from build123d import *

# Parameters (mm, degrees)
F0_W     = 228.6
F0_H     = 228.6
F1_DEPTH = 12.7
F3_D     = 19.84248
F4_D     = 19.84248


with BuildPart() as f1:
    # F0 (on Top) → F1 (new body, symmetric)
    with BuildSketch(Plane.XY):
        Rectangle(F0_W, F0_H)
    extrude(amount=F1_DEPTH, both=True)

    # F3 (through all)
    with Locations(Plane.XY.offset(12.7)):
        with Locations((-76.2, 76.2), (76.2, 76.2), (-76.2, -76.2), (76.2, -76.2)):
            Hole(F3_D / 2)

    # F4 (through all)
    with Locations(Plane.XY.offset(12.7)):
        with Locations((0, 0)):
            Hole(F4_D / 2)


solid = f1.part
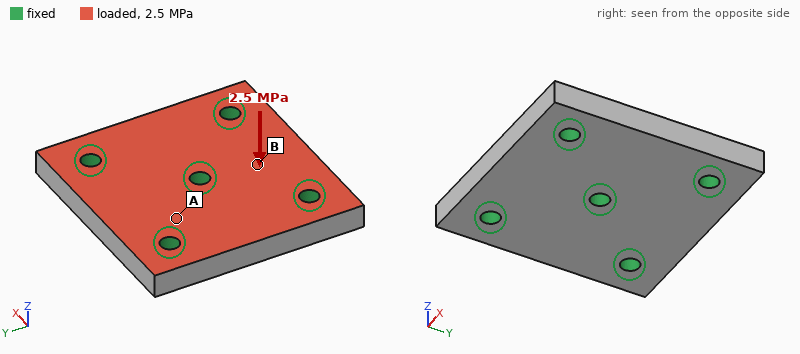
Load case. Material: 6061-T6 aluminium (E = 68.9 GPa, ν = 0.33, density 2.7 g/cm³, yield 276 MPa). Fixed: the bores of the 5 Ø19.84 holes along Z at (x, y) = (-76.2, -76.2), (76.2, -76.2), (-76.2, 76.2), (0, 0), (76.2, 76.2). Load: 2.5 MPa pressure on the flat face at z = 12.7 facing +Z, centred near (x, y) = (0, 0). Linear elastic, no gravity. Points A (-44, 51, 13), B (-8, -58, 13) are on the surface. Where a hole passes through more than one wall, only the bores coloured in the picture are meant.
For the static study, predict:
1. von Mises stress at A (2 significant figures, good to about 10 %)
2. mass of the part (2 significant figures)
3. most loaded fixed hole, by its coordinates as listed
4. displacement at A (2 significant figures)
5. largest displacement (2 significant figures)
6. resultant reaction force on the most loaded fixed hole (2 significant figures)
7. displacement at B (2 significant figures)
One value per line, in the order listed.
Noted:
17 MPa
3.5 kg
(0, 0)
17 µm
47 µm
28 kN
25 µm
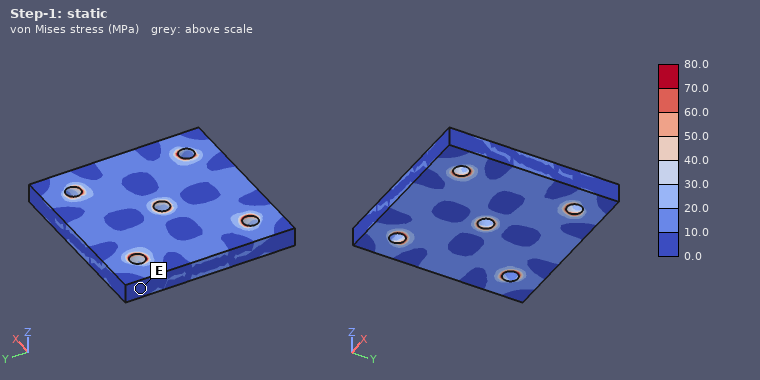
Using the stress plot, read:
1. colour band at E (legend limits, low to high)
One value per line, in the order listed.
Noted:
0.0 to 10.0 MPa
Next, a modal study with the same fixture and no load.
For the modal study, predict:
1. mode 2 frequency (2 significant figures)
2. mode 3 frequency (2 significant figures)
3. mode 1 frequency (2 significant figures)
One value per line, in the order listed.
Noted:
5400 Hz
5400 Hz
5100 Hz
